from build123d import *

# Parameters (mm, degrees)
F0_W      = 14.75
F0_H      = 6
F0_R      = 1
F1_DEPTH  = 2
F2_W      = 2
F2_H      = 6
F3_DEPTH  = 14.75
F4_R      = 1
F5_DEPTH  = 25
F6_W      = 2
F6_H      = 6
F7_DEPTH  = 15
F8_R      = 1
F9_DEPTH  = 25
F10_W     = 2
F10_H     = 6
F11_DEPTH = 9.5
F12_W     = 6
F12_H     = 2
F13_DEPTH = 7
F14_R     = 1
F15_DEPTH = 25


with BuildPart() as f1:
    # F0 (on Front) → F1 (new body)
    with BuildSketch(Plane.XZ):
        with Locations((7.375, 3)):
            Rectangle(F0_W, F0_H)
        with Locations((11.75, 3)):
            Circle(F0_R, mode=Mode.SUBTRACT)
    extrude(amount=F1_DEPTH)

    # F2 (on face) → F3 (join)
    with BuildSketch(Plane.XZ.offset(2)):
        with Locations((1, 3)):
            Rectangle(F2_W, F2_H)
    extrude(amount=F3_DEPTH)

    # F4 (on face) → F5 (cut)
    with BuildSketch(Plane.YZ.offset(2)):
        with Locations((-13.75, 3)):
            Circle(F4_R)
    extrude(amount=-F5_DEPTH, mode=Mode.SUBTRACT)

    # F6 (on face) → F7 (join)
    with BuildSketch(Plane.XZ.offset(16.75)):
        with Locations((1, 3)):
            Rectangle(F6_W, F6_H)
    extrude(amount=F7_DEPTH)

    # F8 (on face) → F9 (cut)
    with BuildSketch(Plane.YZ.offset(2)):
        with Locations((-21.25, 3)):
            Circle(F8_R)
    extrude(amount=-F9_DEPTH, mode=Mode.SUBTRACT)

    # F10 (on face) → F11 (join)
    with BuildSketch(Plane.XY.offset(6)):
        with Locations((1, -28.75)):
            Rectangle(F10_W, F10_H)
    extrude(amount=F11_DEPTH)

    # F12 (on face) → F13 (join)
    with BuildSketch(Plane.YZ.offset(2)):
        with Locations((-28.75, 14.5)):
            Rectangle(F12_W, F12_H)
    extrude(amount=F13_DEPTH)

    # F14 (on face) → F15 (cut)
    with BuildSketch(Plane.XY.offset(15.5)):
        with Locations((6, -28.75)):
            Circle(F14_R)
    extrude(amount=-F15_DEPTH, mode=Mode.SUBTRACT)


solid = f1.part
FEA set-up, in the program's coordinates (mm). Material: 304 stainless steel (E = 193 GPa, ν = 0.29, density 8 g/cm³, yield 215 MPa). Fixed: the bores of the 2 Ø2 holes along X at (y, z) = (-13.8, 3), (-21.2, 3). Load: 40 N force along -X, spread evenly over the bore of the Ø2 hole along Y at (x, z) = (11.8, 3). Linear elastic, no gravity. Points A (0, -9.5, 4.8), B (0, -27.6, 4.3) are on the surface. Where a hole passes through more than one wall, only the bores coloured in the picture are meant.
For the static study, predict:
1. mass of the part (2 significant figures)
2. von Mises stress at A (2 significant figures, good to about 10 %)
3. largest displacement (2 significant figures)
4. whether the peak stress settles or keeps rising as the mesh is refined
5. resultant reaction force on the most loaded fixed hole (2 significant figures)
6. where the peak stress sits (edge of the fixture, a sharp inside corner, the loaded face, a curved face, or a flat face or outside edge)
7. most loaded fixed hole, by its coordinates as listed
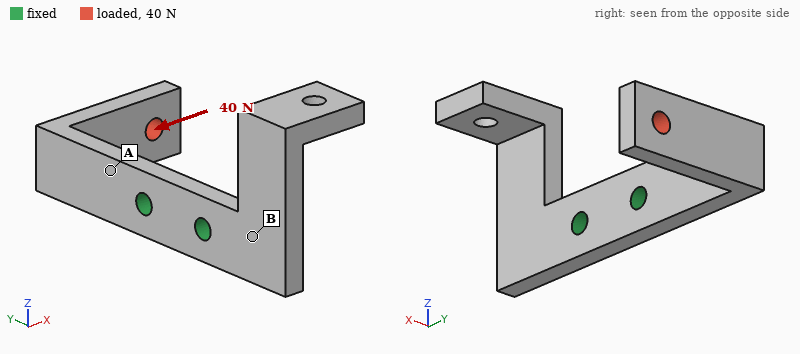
5.7 g
83 MPa
65 µm
keeps rising
47 N
edge of the fixture
(-13.8, 3)
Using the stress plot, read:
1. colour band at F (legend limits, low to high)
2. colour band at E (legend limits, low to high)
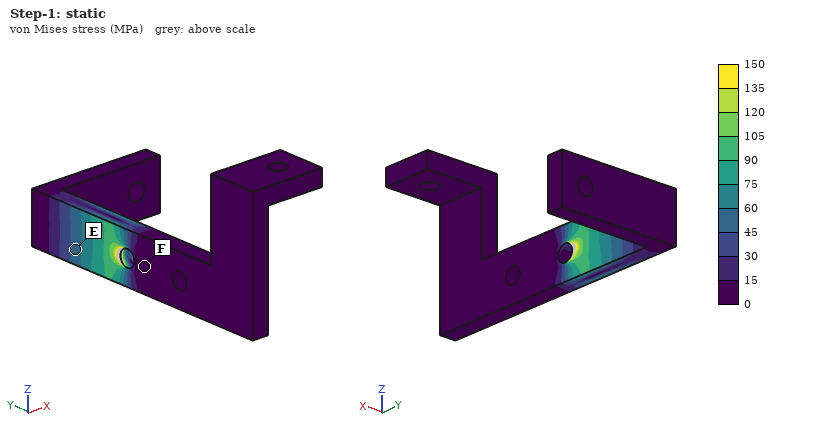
0 to 15 MPa
45 to 60 MPa
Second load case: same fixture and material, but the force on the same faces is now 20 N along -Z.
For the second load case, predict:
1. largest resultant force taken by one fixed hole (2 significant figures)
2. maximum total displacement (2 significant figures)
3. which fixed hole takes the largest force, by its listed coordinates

35 N
40 µm
(-13.8, 3)
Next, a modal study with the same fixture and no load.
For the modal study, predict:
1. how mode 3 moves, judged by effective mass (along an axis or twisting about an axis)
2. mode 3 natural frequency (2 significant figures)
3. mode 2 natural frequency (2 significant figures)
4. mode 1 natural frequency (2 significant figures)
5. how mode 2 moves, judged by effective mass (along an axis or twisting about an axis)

along Z
4700 Hz
3900 Hz
3200 Hz
along X
